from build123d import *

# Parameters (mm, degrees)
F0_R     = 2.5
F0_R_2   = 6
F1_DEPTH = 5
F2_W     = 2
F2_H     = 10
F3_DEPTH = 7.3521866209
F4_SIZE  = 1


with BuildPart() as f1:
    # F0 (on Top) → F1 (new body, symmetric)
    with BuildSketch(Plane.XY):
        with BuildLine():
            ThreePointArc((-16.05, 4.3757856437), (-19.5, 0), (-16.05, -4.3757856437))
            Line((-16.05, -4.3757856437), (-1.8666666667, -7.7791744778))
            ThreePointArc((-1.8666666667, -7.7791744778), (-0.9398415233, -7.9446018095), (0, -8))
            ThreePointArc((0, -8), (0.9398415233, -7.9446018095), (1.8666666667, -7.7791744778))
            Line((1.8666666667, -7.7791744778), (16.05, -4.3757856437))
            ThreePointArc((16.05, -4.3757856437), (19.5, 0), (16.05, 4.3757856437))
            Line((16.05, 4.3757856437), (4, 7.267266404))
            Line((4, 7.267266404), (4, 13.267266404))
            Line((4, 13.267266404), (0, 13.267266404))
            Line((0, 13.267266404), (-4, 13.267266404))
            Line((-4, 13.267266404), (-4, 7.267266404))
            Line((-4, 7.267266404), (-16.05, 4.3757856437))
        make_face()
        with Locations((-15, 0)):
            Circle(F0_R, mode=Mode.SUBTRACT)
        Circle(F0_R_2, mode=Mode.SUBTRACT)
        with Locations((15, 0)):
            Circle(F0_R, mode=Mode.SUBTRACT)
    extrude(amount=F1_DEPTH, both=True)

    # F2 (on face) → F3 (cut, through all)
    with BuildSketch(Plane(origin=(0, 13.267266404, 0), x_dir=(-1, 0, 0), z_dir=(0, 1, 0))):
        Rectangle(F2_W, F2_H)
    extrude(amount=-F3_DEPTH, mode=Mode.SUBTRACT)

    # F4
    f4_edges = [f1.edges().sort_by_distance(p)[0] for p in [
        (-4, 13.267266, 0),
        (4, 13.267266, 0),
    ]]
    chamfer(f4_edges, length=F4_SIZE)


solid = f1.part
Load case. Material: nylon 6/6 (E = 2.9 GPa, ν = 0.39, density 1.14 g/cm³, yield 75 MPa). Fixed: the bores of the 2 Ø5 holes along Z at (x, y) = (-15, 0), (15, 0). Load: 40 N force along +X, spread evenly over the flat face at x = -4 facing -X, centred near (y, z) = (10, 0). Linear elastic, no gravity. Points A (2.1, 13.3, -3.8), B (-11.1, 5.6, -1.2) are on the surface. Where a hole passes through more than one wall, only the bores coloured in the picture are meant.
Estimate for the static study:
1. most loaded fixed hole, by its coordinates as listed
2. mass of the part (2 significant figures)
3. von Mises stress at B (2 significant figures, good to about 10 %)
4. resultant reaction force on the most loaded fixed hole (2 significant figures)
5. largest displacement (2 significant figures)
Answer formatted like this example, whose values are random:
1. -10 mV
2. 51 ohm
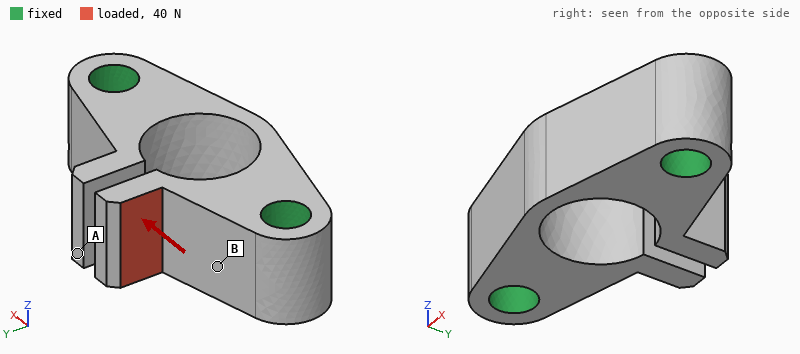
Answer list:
1. (-15, 0)
2. 3.7 g
3. 3.6 MPa
4. 46 N
5. 0.16 mm
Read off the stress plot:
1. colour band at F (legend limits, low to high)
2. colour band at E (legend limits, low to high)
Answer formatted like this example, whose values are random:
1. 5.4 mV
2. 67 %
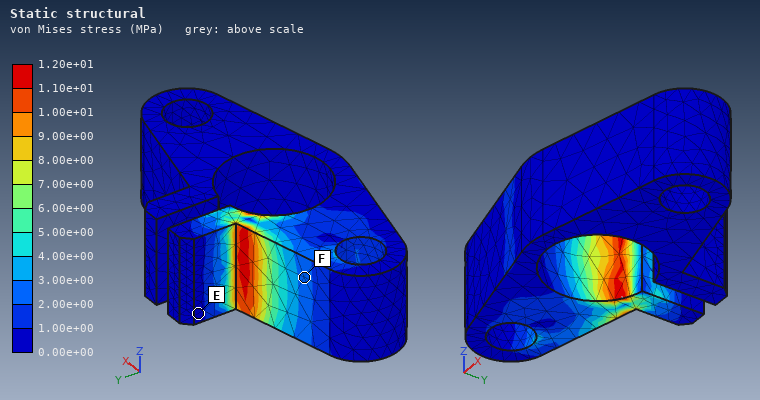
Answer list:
1. 2.00e+00 to 3.00e+00 MPa
2. 0.00e+00 to 1.00e+00 MPa
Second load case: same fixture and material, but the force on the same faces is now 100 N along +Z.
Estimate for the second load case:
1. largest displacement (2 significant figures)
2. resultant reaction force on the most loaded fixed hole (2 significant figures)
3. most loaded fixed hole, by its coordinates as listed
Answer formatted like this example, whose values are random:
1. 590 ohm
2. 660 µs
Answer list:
1. 0.20 mm
2. 100 N
3. (-15, 0)
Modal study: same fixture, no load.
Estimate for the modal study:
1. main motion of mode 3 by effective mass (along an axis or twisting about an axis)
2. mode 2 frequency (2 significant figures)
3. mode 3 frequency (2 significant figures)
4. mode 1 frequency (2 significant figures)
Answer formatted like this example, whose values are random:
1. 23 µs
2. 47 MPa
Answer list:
1. along Z
2. 5700 Hz
3. 8200 Hz
4. 5700 Hz
